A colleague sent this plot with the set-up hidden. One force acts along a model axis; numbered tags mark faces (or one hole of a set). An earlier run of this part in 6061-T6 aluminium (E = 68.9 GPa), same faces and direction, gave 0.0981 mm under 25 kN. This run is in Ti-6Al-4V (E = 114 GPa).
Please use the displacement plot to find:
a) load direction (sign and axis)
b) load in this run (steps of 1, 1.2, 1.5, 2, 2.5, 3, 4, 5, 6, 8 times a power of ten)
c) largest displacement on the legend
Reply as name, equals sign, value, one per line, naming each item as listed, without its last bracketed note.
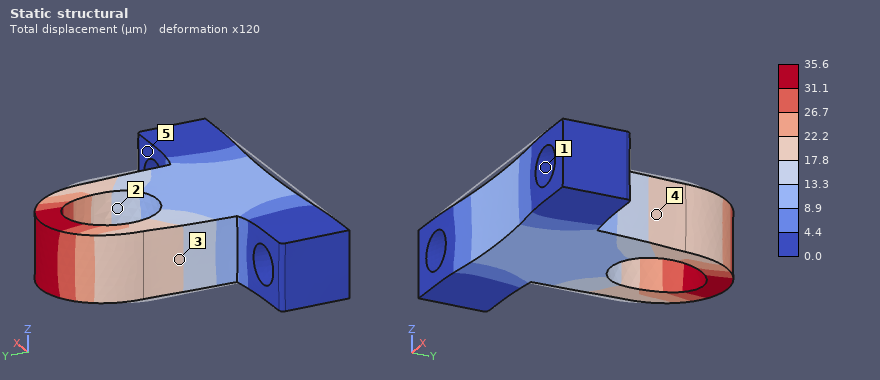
load direction = +Y
load in this run = 15 kN
largest displacement on the legend = 35.6 µm
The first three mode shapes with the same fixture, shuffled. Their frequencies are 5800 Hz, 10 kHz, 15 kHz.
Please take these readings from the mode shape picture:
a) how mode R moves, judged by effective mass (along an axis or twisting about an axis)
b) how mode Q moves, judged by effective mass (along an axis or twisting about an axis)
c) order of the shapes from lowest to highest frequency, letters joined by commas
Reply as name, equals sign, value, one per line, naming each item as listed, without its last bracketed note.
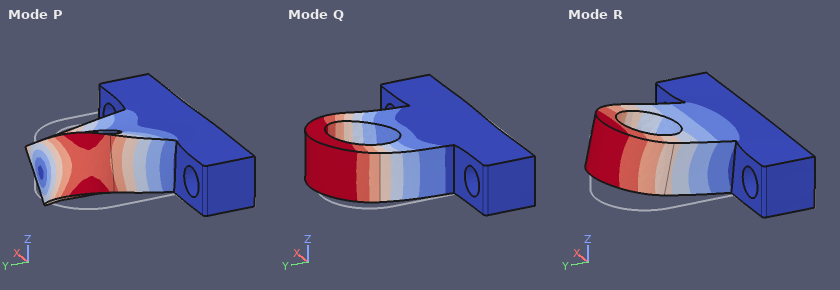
how mode R moves, judged by effective mass = along Z
how mode Q moves, judged by effective mass = along X
order of the shapes from lowest to highest frequency, letters joined by commas = R, Q, P
